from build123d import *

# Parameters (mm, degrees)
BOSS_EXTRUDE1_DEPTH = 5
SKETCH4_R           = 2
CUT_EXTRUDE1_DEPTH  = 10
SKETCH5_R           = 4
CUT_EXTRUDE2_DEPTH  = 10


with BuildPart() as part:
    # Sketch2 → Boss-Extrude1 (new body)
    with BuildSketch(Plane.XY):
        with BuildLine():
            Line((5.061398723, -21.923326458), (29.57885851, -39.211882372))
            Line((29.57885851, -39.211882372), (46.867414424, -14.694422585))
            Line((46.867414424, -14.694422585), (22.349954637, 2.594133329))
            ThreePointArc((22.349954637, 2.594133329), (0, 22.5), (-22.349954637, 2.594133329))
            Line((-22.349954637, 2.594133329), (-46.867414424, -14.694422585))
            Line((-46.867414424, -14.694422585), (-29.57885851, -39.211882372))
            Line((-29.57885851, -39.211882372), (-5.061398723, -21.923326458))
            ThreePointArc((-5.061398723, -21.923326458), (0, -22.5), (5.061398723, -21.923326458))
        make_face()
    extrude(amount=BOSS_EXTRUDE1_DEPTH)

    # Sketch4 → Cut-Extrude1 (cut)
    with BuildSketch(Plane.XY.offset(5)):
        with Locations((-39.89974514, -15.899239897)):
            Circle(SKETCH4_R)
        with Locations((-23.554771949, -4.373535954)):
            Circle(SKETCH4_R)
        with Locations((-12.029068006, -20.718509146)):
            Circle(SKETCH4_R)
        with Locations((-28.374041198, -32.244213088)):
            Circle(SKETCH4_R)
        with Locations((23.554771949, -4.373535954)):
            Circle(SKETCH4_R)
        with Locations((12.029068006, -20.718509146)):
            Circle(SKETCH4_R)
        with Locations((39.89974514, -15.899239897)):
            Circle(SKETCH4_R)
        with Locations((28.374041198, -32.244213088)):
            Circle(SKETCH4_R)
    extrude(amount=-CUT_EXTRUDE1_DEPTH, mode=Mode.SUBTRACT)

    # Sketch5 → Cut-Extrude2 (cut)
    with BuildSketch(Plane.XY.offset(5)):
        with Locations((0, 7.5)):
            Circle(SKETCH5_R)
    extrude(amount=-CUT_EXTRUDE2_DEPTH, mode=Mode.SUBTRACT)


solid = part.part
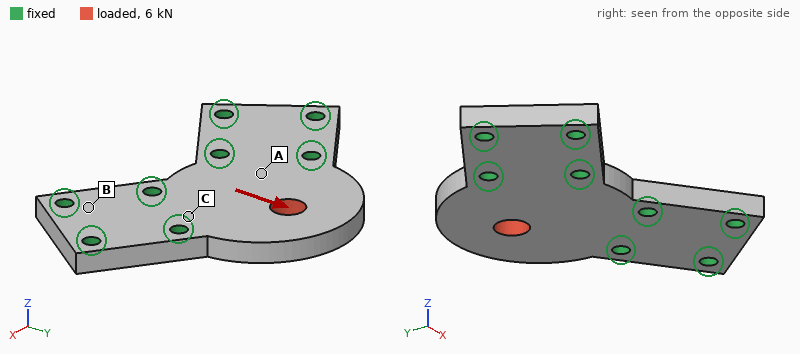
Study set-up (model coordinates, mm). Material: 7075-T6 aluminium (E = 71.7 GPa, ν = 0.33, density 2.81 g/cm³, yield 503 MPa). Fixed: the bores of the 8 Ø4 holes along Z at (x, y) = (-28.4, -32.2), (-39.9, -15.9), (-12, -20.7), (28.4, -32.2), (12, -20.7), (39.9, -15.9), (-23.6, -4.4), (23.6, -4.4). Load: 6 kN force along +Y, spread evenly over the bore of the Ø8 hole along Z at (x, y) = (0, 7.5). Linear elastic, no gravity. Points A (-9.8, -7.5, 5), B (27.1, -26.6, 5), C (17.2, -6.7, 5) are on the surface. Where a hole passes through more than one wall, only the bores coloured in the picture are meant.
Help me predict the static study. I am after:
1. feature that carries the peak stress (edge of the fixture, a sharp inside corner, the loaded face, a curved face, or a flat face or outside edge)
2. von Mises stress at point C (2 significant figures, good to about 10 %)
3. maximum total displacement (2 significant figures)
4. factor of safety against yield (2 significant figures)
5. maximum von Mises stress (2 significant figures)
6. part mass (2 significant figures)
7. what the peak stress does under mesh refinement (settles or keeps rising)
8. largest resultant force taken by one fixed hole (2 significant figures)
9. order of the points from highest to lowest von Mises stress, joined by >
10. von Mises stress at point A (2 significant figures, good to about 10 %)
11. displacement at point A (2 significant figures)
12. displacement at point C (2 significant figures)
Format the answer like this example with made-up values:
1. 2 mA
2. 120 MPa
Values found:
1. the loaded face
2. 18 MPa
3. 18 µm
4. 5.3
5. 95 MPa
6. 42 g
7. settles
8. 1.8 kN
9. A > C > B
10. 28 MPa
11. 5.2 µm
12. 2.8 µm
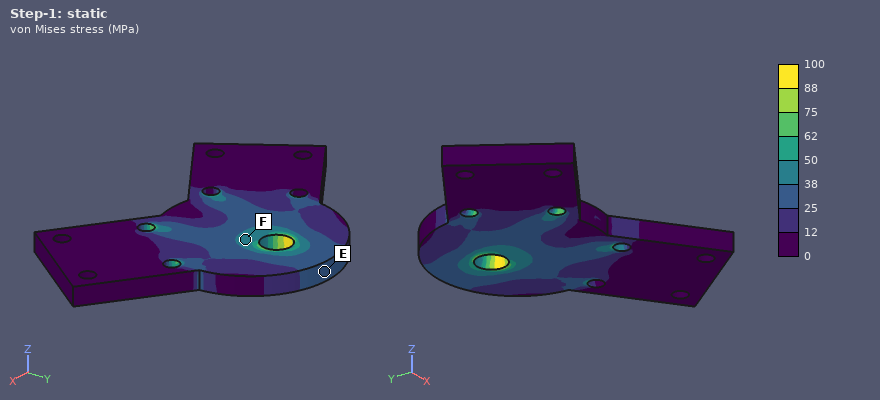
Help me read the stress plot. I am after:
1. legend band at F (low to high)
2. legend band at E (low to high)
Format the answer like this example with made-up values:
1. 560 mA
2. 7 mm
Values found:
1. 38 to 50 MPa
2. 25 to 38 MPa
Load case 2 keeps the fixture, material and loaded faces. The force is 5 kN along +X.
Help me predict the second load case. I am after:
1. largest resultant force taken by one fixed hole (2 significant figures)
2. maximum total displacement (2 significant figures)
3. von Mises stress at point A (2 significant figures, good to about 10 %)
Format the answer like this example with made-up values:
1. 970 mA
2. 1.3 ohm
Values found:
1. 2.2 kN
2. 20 µm
3. 15 MPa
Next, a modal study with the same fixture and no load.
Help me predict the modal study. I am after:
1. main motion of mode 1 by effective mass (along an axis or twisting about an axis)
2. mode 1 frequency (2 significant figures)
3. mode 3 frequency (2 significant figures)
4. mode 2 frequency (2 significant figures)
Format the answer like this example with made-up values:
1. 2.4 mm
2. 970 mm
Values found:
1. along Z
2. 5200 Hz
3. 18 kHz
4. 14 kHz
